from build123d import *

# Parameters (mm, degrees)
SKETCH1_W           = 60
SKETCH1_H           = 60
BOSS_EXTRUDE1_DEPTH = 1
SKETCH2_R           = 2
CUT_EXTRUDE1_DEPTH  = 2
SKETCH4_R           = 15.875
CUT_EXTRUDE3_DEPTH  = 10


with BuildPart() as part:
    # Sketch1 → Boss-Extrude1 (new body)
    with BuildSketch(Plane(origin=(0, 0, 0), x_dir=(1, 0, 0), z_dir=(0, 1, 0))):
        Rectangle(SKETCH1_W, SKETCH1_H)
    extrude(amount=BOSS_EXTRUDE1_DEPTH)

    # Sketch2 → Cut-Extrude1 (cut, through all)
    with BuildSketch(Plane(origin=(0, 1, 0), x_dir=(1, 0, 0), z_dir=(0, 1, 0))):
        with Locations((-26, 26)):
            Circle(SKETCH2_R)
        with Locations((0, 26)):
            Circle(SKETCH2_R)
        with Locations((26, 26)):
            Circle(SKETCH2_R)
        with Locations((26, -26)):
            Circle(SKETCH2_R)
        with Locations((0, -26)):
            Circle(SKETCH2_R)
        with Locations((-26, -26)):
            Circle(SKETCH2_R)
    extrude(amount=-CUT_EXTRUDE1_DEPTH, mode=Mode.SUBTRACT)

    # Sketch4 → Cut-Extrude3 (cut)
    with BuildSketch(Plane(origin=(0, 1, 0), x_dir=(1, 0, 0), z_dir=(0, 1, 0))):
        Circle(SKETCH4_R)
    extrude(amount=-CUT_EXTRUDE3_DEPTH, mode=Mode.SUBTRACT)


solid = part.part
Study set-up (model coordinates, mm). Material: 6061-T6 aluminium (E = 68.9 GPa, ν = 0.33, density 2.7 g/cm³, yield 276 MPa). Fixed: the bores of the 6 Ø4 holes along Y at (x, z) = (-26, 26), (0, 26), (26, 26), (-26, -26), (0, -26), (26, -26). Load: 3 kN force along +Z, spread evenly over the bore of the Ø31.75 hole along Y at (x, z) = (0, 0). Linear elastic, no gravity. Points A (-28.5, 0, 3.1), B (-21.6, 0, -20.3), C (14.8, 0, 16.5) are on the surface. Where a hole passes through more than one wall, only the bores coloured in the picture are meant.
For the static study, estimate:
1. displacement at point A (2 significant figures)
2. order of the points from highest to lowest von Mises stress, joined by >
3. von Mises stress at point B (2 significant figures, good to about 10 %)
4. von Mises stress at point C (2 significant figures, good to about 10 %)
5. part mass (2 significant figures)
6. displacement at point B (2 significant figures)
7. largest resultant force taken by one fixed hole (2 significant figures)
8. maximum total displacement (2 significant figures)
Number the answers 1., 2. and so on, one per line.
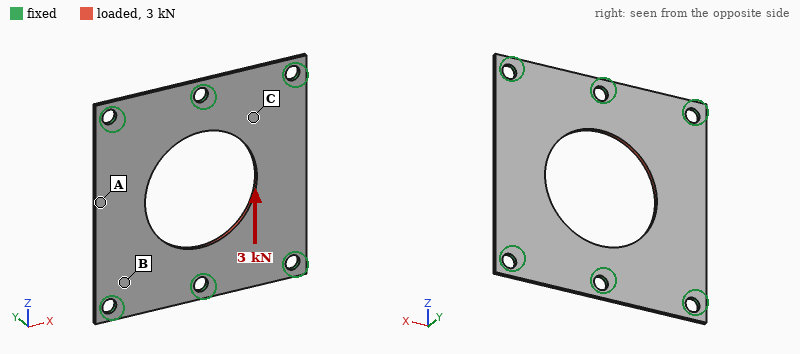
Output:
1. 5.4 µm
2. B > C > A
3. 39 MPa
4. 25 MPa
5. 7.4 g
6. 4.2 µm
7. 700 N
8. 13 µm
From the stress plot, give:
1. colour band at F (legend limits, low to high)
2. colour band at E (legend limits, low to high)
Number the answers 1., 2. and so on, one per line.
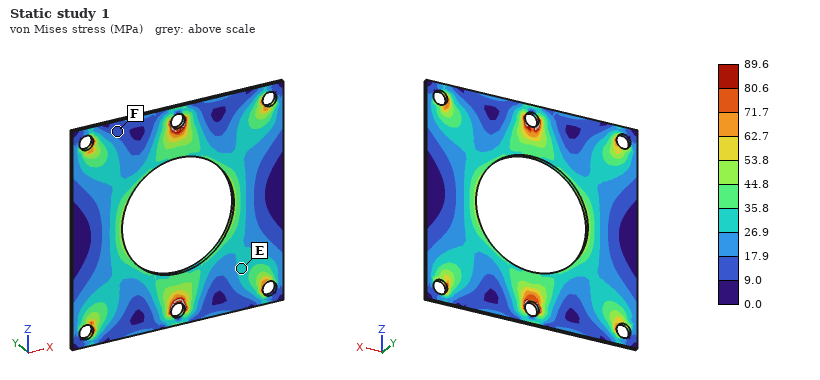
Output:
1. 9.0 to 17.9 MPa
2. 26.9 to 35.8 MPa
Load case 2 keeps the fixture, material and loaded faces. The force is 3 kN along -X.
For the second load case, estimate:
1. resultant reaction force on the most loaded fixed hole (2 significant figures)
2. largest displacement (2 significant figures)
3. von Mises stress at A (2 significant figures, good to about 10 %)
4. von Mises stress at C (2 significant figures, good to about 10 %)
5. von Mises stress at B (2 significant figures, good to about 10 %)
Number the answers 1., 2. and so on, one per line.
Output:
1. 780 N
2. 29 µm
3. 37 MPa
4. 42 MPa
5. 44 MPa
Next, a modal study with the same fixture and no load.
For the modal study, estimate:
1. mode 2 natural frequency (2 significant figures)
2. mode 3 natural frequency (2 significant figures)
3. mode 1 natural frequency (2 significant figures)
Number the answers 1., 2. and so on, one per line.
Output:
1. 2300 Hz
2. 4900 Hz
3. 2200 Hz
